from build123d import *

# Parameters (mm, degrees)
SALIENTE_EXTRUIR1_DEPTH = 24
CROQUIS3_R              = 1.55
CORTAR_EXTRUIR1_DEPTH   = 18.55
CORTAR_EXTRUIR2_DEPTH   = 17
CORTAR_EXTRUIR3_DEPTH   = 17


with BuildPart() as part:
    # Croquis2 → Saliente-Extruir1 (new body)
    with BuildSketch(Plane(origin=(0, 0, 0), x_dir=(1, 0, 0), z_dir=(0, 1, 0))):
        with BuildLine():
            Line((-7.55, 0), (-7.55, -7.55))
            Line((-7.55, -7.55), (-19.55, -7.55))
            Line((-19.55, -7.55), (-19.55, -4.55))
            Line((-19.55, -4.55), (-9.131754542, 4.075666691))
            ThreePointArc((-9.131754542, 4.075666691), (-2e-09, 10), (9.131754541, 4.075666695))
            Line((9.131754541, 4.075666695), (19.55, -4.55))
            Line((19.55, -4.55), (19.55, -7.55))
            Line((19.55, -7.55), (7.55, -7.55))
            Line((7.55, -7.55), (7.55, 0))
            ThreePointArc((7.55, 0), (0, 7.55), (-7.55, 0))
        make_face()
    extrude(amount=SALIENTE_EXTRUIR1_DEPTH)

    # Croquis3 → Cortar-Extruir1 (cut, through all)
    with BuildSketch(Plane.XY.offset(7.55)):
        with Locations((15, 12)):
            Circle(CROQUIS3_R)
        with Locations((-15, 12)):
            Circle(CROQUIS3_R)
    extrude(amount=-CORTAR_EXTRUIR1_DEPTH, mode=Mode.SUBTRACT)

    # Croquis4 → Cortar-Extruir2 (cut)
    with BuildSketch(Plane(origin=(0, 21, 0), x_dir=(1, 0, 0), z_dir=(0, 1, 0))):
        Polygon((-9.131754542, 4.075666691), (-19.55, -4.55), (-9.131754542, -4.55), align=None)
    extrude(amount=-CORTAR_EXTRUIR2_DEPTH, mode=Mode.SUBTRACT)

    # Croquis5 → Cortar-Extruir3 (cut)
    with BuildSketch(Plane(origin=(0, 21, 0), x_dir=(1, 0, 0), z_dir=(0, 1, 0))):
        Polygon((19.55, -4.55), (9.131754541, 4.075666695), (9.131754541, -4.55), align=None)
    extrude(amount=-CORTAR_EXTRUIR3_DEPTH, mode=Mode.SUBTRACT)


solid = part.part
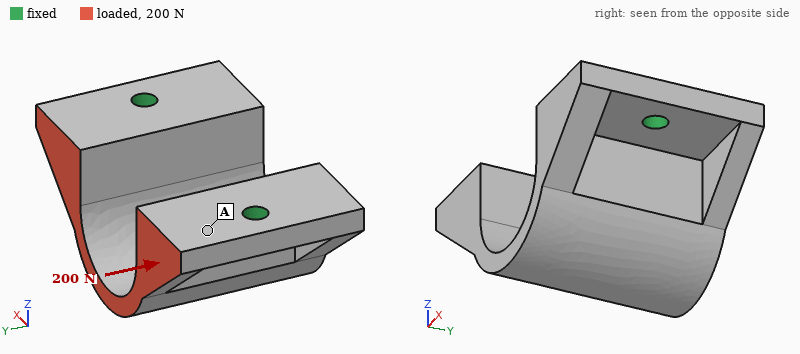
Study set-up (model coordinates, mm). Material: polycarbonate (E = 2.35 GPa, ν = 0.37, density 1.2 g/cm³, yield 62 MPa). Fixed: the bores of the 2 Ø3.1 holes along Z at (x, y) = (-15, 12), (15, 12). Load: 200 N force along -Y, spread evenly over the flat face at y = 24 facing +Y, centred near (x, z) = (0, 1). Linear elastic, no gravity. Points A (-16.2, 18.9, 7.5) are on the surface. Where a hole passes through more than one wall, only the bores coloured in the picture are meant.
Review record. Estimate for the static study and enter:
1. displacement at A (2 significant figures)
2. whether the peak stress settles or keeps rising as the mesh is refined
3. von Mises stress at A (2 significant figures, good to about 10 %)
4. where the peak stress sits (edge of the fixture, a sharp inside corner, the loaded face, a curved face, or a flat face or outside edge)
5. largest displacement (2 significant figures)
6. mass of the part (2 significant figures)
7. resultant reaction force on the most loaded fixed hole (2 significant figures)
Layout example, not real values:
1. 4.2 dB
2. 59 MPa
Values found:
1. 0.086 mm
2. keeps rising
3. 4.9 MPa
4. edge of the fixture
5. 0.42 mm
6. 5.0 g
7. 100 N
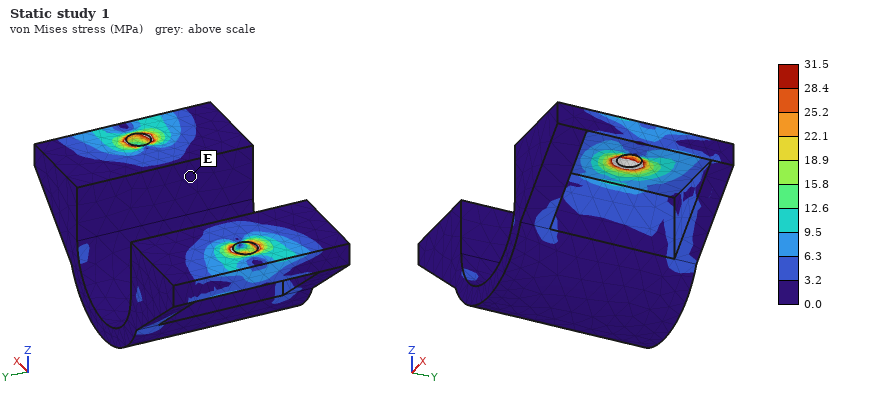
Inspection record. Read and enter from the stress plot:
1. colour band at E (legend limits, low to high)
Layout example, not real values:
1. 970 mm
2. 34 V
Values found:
1. 0.0 to 3.2 MPa
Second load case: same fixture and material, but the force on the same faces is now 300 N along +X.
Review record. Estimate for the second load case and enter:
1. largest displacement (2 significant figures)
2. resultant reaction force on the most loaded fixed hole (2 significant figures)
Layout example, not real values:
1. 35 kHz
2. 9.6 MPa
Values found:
1. 0.55 mm
2. 160 N
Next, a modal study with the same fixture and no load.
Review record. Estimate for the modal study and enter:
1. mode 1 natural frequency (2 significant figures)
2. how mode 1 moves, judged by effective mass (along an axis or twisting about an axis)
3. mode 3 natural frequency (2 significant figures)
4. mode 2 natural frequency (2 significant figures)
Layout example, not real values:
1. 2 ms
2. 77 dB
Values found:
1. 1600 Hz
2. along Y
3. 3200 Hz
4. 3100 Hz
